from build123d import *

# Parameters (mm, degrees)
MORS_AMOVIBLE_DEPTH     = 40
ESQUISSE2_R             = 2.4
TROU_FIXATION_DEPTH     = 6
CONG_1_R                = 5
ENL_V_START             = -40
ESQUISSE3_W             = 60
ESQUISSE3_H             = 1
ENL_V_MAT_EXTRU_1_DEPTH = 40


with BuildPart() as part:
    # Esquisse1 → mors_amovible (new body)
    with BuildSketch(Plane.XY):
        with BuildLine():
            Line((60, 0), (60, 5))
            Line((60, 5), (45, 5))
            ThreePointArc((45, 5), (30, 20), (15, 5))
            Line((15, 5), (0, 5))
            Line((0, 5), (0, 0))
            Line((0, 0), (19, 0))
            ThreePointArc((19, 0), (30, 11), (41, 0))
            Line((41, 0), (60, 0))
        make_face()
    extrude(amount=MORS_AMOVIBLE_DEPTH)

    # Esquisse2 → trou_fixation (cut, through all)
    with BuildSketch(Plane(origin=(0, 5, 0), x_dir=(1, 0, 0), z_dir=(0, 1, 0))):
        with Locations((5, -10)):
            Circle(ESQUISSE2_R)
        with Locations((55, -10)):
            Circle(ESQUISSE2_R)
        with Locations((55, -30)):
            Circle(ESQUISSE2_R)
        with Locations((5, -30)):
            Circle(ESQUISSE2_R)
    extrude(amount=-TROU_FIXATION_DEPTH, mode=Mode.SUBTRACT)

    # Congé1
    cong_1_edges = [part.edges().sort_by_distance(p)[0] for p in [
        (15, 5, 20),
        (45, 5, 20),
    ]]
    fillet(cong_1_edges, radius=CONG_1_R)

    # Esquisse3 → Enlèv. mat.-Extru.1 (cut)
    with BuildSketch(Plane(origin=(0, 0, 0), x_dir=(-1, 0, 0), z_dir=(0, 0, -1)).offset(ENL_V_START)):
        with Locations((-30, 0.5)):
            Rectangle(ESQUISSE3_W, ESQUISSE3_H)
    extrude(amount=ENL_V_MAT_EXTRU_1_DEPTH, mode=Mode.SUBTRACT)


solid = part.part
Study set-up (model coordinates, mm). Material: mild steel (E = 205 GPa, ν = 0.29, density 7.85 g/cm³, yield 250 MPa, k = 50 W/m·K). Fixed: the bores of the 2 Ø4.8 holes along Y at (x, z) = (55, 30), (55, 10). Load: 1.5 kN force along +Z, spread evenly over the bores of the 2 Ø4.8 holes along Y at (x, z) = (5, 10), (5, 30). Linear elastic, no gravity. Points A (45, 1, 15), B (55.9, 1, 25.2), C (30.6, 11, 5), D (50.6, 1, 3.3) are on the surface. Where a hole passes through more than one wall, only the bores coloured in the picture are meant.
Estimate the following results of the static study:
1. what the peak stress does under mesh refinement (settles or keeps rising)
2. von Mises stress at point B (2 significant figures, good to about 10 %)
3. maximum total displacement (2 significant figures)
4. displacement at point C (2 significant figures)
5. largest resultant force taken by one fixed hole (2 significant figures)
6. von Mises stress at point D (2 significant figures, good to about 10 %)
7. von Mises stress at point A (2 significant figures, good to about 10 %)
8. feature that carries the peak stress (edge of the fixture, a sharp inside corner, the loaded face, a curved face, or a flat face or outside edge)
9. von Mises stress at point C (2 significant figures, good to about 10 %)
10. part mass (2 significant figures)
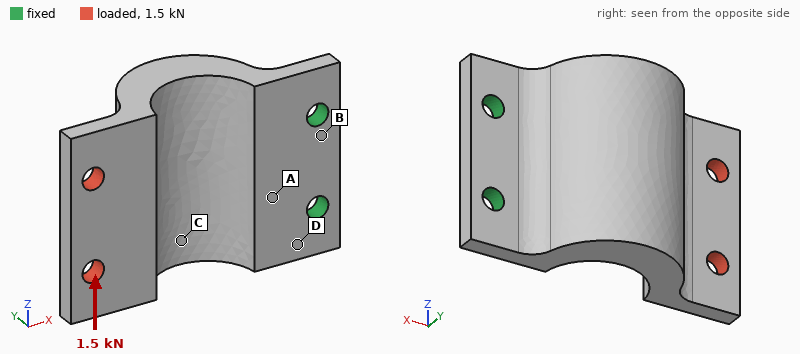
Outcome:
keeps rising
13 MPa
92 µm
34 µm
3.2 kN
26 MPa
100 MPa
edge of the fixture
87 MPa
130 g
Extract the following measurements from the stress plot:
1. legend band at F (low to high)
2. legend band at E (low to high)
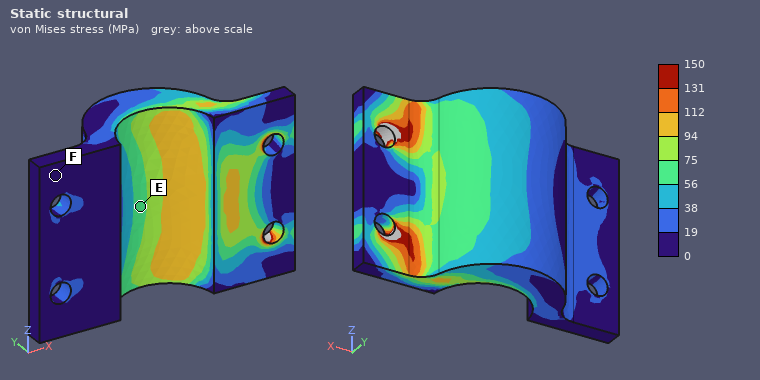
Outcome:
0 to 19 MPa
56 to 75 MPa
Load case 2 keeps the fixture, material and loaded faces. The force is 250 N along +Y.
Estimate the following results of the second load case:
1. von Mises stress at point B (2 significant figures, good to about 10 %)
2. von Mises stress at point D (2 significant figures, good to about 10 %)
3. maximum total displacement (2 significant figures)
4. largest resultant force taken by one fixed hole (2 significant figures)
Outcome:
35 MPa
83 MPa
0.15 mm
130 N
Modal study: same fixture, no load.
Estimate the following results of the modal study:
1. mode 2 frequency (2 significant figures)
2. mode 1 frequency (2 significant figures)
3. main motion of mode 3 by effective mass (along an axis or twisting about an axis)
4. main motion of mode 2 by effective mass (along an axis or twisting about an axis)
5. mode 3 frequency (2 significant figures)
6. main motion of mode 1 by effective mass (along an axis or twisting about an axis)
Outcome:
3600 Hz
1100 Hz
along Z
along Z
5600 Hz
along Y
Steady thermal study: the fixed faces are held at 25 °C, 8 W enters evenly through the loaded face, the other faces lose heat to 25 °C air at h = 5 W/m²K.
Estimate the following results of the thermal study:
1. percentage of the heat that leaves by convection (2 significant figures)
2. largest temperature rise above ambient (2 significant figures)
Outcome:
8.3 %
43 K
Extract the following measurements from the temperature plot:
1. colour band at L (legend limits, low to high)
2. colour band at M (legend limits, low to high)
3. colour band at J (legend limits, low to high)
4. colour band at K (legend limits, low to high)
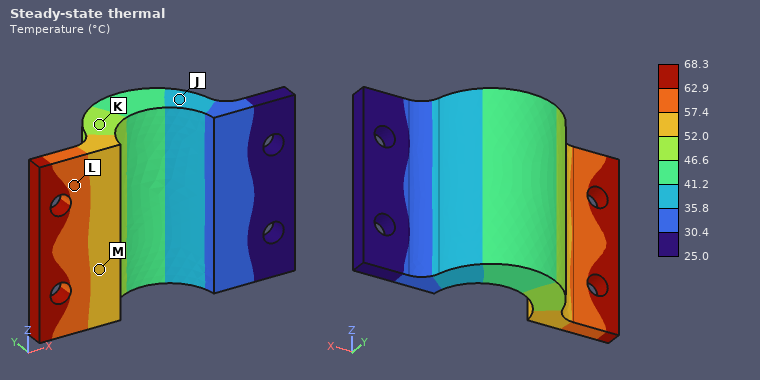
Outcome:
57.4 to 62.9 °C
52.0 to 57.4 °C
35.8 to 41.2 °C
46.6 to 52.0 °C
